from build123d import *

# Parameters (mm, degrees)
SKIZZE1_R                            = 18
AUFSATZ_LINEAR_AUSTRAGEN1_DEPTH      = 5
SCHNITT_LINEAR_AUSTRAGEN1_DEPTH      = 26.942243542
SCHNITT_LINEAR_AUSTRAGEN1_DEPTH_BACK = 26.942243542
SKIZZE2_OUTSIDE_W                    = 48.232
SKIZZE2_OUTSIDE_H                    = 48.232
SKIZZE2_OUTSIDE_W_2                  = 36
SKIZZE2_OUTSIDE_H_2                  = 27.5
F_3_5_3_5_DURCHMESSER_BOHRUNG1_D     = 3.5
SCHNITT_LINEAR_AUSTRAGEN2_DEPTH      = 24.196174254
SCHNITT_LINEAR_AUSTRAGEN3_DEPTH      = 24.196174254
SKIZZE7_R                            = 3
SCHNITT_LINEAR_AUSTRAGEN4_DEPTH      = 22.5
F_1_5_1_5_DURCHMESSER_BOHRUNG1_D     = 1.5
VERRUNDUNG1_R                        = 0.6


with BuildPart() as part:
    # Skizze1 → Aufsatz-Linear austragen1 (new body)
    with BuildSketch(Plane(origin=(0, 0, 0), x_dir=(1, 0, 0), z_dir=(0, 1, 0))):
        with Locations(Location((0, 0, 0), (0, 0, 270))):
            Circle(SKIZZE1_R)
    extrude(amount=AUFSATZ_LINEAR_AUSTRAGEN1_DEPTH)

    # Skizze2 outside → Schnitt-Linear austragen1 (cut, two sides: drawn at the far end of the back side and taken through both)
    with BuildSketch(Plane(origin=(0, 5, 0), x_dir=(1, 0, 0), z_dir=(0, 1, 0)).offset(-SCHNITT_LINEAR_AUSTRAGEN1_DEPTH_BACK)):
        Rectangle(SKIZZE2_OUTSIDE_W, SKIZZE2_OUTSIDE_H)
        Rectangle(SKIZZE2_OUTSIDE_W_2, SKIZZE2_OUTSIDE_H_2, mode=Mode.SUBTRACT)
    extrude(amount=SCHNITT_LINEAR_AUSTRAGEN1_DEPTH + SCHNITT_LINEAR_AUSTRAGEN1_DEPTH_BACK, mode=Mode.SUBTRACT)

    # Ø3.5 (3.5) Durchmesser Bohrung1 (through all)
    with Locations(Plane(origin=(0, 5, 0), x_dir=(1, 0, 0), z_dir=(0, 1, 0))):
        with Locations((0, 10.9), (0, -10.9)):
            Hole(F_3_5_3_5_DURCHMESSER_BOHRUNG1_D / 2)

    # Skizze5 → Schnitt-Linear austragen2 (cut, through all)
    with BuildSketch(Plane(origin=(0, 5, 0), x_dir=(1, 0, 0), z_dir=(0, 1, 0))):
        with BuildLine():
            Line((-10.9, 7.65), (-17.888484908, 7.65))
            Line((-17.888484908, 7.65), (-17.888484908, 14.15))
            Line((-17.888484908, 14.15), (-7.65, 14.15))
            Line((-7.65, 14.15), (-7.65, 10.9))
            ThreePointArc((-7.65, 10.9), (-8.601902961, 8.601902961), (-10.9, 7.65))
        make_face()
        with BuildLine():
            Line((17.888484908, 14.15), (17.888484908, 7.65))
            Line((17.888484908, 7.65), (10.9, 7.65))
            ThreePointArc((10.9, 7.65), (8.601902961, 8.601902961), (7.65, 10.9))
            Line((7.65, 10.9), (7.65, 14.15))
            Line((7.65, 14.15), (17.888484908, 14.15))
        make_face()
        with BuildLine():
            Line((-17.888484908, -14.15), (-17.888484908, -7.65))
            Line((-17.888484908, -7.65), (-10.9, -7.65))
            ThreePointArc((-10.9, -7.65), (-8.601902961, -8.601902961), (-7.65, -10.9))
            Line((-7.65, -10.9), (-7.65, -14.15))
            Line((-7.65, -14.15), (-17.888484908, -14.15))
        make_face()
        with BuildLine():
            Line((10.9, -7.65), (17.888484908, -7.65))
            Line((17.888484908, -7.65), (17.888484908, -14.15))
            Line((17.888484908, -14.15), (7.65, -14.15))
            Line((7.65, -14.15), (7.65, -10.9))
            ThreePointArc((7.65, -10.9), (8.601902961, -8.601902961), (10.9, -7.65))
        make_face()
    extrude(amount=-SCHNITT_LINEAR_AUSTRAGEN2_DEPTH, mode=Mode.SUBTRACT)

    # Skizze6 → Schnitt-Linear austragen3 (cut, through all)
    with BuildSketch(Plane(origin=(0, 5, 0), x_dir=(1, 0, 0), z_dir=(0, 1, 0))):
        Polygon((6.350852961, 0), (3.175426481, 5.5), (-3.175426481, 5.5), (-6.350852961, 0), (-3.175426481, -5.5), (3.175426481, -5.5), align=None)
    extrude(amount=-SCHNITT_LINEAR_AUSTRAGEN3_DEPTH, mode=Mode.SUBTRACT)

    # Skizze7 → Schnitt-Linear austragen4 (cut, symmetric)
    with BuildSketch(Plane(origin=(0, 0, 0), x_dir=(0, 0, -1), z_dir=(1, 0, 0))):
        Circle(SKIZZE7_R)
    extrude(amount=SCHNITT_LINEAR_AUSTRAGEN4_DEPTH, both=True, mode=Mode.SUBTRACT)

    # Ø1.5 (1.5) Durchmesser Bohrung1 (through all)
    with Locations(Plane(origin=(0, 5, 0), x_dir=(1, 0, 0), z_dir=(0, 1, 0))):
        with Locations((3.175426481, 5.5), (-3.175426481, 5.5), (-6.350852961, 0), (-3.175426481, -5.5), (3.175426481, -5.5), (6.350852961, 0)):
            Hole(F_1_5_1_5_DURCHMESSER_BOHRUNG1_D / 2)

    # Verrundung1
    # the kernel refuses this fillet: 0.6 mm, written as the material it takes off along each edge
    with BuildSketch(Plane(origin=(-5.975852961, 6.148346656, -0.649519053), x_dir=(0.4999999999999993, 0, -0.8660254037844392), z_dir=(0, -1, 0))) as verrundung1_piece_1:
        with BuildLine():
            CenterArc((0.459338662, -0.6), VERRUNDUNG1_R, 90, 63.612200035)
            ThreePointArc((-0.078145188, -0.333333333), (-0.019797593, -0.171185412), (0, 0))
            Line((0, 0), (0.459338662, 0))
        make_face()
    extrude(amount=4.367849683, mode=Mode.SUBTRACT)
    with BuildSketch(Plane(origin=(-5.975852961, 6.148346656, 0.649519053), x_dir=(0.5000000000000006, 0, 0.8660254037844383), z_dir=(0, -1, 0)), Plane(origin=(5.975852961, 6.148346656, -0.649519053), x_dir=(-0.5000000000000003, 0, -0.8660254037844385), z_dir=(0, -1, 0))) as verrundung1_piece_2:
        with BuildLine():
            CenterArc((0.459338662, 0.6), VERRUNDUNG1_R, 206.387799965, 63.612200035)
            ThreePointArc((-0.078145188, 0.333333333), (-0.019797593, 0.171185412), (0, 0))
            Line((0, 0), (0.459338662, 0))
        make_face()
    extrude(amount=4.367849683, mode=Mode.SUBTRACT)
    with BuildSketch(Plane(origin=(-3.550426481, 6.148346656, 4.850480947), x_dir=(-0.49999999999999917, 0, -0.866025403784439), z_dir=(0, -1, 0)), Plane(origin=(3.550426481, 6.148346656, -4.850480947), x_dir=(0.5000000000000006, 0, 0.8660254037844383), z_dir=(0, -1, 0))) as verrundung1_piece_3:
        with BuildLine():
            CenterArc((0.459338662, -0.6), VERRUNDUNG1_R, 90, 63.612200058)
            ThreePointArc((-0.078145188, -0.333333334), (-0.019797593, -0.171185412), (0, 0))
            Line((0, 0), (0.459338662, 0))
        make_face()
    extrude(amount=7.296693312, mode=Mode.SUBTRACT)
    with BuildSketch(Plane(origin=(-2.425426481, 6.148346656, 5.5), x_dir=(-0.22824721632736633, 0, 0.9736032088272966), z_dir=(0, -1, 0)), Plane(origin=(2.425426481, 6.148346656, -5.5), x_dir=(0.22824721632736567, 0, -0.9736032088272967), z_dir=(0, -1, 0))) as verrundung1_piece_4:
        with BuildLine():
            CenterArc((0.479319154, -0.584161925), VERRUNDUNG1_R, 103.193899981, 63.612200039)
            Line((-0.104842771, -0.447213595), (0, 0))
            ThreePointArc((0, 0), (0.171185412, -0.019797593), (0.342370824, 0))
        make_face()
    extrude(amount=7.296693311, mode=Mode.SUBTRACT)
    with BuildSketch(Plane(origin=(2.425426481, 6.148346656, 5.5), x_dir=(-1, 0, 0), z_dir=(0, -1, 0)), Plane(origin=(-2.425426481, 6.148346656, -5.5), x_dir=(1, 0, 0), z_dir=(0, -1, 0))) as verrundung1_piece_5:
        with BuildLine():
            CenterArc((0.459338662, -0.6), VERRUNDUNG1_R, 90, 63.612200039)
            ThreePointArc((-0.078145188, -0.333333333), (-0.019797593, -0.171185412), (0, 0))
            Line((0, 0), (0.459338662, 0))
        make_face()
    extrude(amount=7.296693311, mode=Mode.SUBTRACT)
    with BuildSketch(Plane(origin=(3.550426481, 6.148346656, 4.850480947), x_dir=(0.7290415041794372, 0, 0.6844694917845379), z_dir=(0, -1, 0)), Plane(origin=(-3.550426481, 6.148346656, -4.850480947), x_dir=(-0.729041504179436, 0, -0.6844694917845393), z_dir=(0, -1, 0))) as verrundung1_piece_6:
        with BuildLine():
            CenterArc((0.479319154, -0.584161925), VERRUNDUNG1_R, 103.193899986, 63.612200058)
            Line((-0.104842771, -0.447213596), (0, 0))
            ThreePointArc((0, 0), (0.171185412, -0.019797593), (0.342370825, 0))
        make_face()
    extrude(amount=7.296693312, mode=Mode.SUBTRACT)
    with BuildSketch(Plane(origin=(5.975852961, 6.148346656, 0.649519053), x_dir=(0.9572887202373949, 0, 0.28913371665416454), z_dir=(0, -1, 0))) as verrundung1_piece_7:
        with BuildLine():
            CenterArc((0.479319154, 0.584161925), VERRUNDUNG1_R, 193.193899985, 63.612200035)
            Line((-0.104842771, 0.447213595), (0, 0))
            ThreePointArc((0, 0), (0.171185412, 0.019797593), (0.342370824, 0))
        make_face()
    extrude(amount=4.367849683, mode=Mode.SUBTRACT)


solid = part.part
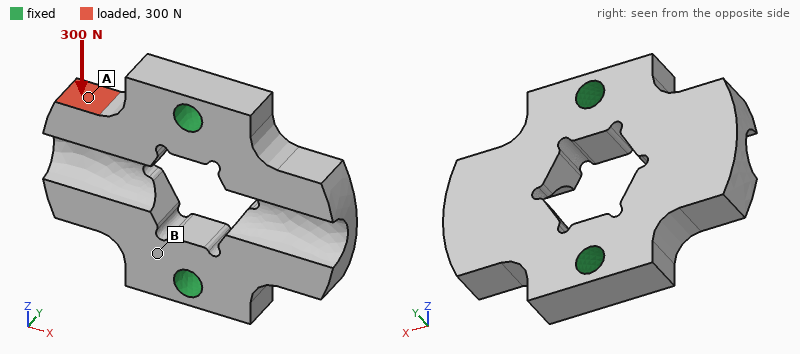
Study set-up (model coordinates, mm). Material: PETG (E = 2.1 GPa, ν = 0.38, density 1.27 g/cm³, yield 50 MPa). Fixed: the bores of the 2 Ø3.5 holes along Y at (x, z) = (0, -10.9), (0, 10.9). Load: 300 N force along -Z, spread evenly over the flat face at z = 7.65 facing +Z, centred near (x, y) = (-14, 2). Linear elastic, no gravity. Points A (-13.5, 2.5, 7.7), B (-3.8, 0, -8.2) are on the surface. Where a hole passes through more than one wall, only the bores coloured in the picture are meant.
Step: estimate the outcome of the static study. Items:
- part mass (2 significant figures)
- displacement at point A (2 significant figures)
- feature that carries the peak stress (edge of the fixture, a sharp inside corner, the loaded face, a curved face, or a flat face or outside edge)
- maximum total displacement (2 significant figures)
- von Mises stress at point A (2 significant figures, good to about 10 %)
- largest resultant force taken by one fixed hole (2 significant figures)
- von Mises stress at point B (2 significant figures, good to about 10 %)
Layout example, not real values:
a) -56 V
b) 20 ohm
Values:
a) 3.4 g
b) 0.17 mm
c) a curved face
d) 0.26 mm
e) 12 MPa
f) 220 N
g) 4.9 MPa
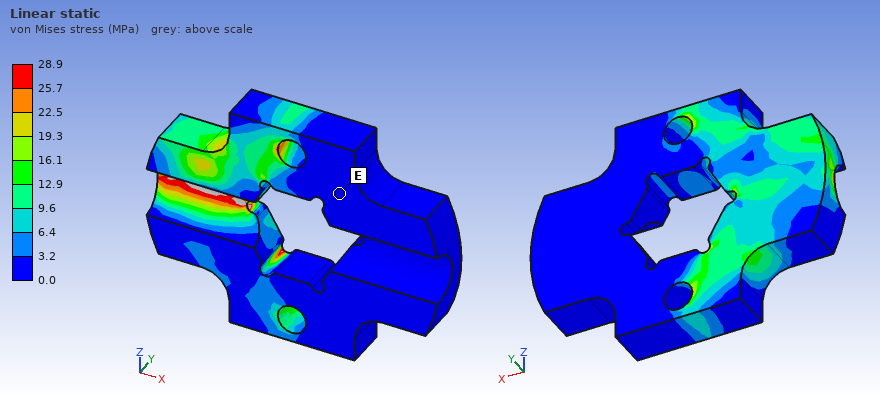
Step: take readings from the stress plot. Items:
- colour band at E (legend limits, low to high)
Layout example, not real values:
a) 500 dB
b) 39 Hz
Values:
a) 0.0 to 3.2 MPa
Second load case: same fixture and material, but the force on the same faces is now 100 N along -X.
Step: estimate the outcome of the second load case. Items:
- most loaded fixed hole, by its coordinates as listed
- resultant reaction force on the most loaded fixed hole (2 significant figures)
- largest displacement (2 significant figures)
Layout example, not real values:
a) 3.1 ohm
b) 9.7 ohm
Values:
a) (0, 10.9)
b) 94 N
c) 55 µm
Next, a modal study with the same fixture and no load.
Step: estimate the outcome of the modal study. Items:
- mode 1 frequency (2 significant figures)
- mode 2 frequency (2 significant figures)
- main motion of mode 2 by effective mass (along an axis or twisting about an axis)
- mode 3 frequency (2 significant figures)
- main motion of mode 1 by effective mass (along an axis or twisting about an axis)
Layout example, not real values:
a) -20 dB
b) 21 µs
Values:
a) 3100 Hz
b) 3200 Hz
c) along Y
d) 6900 Hz
e) twisting about Z
